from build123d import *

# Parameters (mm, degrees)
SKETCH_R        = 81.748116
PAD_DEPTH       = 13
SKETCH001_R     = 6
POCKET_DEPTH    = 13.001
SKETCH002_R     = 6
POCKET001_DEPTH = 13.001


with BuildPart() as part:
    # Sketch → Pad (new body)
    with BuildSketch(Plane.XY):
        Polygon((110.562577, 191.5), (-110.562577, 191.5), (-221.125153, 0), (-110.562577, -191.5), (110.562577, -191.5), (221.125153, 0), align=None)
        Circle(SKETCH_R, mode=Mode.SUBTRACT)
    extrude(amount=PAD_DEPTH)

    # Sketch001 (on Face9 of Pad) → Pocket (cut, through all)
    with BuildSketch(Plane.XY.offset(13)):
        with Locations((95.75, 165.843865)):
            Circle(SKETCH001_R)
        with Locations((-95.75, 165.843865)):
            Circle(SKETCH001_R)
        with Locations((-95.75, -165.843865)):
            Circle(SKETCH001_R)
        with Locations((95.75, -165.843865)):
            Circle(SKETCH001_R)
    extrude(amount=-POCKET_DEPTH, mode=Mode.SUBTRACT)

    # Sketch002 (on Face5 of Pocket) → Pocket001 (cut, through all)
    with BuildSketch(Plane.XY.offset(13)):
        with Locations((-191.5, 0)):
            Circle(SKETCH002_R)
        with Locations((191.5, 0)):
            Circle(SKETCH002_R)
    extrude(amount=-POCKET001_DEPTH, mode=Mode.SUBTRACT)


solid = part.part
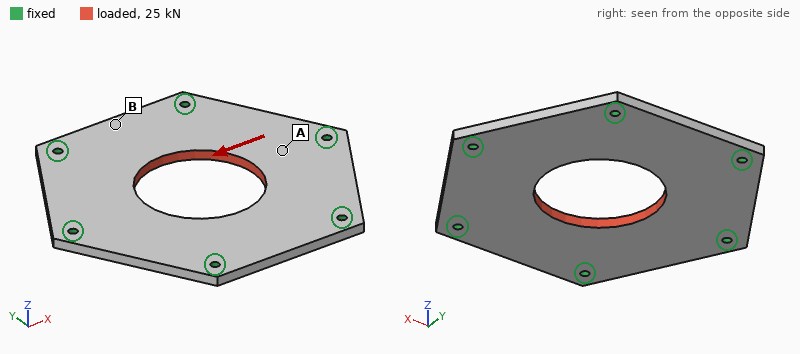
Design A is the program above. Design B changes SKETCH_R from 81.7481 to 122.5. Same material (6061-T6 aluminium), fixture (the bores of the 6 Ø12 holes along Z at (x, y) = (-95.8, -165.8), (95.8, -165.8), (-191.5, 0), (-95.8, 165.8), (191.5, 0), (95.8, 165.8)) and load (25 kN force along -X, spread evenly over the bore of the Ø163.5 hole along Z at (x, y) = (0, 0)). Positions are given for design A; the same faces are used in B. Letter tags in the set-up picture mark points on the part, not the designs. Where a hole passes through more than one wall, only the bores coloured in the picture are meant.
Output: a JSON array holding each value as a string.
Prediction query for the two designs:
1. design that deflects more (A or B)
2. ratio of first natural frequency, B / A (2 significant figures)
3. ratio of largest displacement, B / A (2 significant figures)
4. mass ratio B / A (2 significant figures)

["A", "1.7", "0.92", "0.75"]
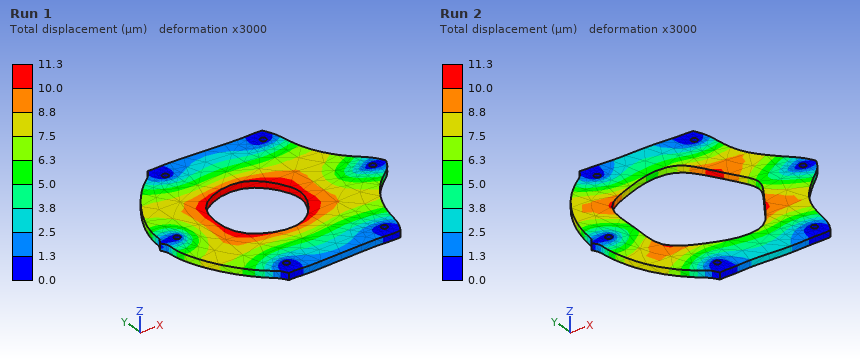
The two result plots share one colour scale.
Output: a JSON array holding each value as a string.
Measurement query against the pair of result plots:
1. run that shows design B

["Run 2"]
